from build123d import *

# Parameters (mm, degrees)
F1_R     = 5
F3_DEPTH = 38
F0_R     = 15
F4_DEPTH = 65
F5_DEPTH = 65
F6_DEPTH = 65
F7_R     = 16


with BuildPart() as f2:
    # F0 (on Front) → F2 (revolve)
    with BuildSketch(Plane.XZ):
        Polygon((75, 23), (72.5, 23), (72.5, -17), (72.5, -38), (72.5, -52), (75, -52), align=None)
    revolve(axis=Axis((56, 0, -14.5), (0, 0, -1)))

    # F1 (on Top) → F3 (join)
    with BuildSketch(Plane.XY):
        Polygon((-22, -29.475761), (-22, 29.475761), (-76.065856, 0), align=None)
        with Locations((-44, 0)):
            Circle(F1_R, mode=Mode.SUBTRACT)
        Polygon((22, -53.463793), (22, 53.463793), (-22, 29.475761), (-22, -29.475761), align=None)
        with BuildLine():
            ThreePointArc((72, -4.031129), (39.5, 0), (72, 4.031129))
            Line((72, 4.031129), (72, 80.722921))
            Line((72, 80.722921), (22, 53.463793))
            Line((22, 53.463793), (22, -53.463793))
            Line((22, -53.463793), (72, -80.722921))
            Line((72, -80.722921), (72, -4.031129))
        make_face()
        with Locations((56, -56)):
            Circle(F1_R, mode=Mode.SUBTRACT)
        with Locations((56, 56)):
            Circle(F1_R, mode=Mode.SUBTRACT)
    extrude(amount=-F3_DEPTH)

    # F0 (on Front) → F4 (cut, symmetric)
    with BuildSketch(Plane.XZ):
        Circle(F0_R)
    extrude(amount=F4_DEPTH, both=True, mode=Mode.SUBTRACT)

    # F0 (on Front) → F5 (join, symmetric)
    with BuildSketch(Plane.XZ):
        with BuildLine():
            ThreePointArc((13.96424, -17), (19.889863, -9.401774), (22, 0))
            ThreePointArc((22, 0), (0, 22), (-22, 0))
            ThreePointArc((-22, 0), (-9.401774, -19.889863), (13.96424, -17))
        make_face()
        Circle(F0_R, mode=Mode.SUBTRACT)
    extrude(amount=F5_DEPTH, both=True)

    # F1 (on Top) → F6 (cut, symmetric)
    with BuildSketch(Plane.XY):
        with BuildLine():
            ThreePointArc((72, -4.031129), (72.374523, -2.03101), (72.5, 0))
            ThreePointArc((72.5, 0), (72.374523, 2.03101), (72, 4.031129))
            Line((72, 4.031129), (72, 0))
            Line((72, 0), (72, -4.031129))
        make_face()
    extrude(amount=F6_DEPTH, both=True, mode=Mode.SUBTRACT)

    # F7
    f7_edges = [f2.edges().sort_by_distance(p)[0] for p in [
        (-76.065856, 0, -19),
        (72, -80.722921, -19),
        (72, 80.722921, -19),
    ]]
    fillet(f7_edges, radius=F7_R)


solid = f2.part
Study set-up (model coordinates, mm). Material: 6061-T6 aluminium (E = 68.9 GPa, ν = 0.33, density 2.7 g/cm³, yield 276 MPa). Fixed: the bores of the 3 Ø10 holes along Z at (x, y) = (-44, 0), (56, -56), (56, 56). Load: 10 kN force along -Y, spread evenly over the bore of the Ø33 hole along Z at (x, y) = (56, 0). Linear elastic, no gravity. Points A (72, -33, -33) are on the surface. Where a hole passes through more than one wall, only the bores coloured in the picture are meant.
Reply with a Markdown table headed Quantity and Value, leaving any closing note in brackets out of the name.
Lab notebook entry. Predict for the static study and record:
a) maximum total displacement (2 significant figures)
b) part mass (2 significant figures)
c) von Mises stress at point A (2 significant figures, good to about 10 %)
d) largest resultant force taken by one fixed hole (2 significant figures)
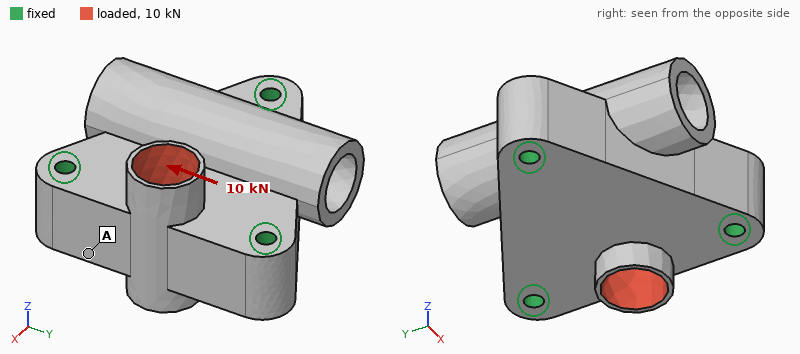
| Quantity | Value |
|---|---|
| maximum total displacement | 19 µm |
| part mass | 1.2 kg |
| von Mises stress at point A | 4.2 MPa |
| largest resultant force taken by one fixed hole | 4.9 kN |
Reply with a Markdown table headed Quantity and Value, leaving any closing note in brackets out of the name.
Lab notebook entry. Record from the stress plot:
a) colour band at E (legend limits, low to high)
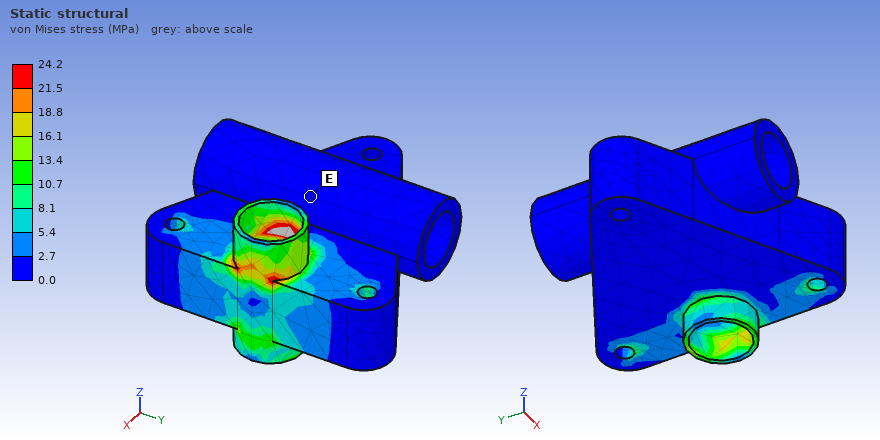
| Quantity | Value |
|---|---|
| colour band at E | 0.0 to 2.7 MPa |
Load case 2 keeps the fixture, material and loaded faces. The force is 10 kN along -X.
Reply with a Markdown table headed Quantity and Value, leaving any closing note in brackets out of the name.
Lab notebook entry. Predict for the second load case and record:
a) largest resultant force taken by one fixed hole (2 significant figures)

| Quantity | Value |
|---|---|
| largest resultant force taken by one fixed hole | 3.5 kN |
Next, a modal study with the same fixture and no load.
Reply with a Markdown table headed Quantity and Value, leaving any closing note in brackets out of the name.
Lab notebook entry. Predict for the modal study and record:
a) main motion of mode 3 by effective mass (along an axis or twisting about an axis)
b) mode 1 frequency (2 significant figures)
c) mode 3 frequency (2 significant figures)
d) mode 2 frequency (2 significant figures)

| Quantity | Value |
|---|---|
| main motion of mode 3 by effective mass | along X |
| mode 1 frequency | 7100 Hz |
| mode 3 frequency | 9100 Hz |
| mode 2 frequency | 7300 Hz |
